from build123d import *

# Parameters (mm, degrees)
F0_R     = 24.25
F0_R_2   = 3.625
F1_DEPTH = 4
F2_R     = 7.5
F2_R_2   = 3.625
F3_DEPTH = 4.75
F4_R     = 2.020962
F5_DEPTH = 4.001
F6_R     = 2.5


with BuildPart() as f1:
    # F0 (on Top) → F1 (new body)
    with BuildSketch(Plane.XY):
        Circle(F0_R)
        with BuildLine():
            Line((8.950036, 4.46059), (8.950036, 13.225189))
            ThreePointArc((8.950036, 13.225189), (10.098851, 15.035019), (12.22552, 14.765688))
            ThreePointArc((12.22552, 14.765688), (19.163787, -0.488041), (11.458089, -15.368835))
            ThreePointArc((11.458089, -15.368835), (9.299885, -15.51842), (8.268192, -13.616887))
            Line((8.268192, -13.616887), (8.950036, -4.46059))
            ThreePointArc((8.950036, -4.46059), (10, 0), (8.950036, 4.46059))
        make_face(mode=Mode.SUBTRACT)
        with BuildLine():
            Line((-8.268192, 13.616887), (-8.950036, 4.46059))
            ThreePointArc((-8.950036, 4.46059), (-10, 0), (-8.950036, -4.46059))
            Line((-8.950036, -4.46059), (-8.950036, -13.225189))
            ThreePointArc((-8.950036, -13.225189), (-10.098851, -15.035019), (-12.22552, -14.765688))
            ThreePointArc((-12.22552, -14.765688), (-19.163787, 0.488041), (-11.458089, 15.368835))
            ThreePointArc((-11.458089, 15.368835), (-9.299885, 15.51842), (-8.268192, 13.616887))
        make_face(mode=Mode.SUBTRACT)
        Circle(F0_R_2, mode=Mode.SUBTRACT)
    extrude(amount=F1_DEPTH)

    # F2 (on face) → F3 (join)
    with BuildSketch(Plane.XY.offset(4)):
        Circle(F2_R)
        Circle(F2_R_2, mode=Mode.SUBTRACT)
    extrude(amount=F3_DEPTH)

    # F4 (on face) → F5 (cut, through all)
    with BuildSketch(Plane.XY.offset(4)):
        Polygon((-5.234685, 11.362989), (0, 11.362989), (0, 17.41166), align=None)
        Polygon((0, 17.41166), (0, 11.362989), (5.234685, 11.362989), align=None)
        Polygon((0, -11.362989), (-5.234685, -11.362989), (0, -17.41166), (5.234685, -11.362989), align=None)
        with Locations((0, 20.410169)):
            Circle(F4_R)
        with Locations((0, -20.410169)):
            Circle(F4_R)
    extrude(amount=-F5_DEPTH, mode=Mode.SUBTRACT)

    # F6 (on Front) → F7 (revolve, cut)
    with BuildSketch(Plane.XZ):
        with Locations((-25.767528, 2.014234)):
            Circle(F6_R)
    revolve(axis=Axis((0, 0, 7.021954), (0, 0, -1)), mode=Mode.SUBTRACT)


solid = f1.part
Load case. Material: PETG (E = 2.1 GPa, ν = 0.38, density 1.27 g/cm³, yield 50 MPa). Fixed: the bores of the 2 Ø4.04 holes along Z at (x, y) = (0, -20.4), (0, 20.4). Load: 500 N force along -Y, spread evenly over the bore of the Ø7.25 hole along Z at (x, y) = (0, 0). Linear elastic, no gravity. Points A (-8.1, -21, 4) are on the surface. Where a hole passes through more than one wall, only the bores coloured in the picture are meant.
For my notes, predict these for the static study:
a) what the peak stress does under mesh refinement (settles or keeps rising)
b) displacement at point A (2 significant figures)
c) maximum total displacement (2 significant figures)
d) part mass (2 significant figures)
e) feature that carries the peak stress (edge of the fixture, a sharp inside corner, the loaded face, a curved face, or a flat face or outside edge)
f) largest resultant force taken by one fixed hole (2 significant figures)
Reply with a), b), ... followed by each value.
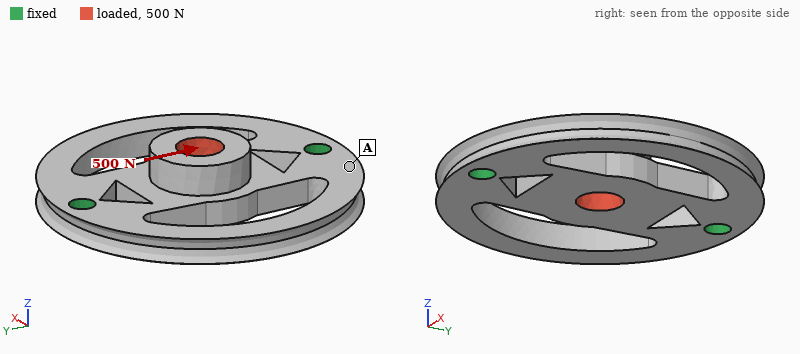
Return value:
a) keeps rising
b) 0.039 mm
c) 0.16 mm
d) 6.6 g
e) a sharp inside corner
f) 250 N
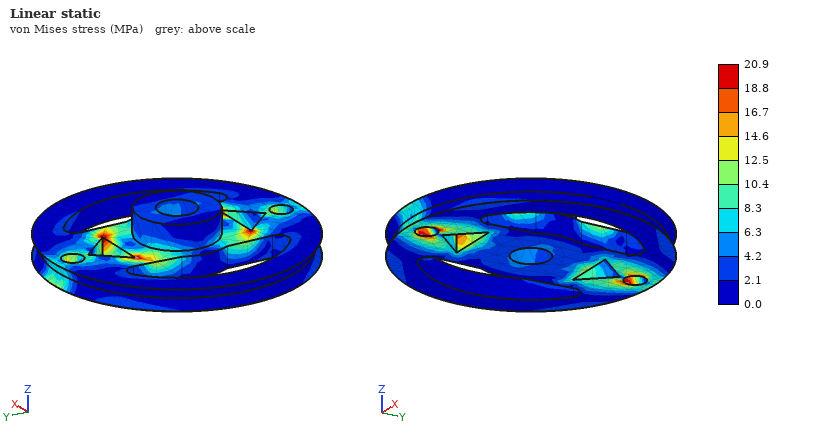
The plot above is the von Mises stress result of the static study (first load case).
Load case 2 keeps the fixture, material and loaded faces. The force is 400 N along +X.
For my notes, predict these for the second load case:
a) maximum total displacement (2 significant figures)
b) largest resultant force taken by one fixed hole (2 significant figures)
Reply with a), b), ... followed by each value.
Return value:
a) 0.44 mm
b) 200 N
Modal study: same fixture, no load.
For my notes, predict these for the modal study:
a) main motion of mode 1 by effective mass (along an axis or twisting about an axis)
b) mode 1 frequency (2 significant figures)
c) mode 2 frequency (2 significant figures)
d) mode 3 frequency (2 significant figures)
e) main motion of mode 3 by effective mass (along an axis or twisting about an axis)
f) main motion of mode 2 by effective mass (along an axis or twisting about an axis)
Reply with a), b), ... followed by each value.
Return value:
a) twisting about Y
b) 1300 Hz
c) 1300 Hz
d) 2600 Hz
e) along Z
f) along Z
